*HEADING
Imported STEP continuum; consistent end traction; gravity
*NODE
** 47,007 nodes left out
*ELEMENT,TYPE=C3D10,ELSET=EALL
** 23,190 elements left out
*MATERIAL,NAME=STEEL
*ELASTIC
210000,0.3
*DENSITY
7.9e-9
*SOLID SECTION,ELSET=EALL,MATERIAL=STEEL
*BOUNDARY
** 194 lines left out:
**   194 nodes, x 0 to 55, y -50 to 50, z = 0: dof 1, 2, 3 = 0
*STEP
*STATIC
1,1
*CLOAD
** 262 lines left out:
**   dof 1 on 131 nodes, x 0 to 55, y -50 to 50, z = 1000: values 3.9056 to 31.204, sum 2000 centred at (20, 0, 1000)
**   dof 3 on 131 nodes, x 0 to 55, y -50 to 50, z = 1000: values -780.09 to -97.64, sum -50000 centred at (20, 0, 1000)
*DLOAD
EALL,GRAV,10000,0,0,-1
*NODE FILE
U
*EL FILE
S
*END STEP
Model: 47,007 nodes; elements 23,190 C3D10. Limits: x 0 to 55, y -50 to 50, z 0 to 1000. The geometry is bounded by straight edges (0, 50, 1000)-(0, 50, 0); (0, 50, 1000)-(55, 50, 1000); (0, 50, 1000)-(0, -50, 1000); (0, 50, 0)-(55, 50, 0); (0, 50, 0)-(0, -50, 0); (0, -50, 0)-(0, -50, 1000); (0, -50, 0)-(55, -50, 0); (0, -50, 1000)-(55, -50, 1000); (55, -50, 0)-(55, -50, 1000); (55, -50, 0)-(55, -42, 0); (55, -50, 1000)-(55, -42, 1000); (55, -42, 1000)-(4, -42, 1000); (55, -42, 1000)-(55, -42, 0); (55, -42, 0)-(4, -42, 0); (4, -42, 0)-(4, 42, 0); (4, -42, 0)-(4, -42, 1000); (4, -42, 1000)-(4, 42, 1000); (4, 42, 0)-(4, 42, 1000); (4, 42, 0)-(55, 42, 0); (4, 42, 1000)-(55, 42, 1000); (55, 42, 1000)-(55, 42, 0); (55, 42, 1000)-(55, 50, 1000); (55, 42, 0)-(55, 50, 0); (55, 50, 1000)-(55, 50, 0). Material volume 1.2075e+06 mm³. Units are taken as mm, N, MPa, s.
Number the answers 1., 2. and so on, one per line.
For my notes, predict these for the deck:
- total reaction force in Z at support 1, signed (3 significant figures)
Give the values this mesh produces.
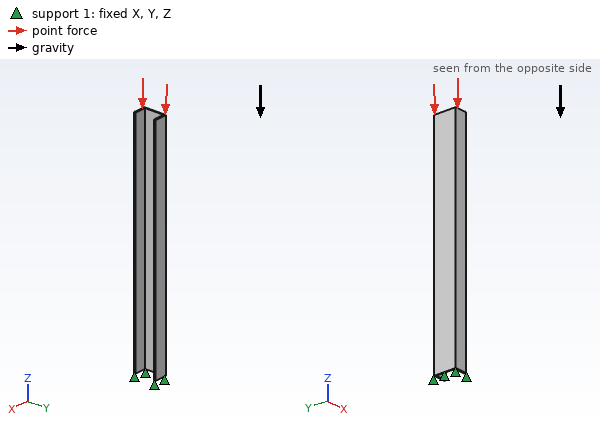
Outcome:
1. 50100 N
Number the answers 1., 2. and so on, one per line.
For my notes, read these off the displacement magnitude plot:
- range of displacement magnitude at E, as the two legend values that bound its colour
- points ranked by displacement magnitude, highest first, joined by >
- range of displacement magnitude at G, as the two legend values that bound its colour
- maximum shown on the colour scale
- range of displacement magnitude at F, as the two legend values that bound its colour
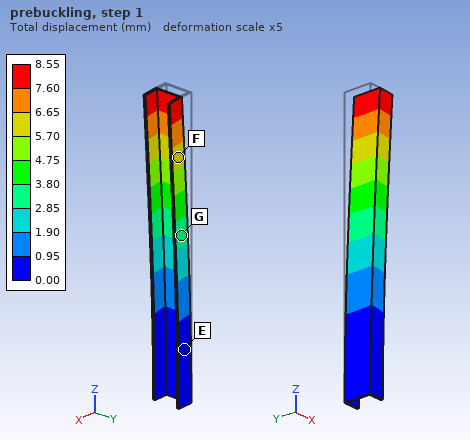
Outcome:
1. 0.00 to 0.95 mm
2. F > G > E
3. 2.85 to 3.80 mm
4. 8.55 mm
5. 5.70 to 6.65 mm
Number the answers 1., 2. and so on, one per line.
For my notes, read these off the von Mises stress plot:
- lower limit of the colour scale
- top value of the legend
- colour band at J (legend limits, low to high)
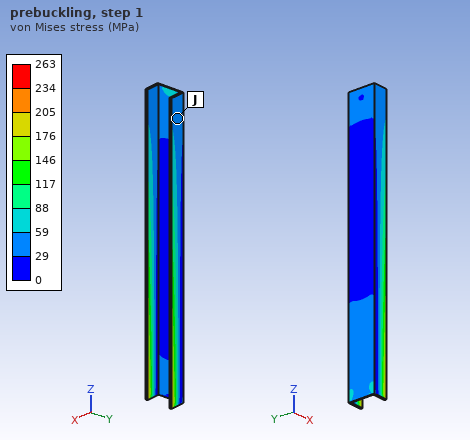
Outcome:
1. 0 MPa
2. 263 MPa
3. 29 to 59 MPa
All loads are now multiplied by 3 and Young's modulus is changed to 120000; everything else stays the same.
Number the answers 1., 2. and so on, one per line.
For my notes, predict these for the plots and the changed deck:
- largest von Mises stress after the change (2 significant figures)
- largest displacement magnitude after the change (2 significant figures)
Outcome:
1. 790 MPa
2. 45 mm
